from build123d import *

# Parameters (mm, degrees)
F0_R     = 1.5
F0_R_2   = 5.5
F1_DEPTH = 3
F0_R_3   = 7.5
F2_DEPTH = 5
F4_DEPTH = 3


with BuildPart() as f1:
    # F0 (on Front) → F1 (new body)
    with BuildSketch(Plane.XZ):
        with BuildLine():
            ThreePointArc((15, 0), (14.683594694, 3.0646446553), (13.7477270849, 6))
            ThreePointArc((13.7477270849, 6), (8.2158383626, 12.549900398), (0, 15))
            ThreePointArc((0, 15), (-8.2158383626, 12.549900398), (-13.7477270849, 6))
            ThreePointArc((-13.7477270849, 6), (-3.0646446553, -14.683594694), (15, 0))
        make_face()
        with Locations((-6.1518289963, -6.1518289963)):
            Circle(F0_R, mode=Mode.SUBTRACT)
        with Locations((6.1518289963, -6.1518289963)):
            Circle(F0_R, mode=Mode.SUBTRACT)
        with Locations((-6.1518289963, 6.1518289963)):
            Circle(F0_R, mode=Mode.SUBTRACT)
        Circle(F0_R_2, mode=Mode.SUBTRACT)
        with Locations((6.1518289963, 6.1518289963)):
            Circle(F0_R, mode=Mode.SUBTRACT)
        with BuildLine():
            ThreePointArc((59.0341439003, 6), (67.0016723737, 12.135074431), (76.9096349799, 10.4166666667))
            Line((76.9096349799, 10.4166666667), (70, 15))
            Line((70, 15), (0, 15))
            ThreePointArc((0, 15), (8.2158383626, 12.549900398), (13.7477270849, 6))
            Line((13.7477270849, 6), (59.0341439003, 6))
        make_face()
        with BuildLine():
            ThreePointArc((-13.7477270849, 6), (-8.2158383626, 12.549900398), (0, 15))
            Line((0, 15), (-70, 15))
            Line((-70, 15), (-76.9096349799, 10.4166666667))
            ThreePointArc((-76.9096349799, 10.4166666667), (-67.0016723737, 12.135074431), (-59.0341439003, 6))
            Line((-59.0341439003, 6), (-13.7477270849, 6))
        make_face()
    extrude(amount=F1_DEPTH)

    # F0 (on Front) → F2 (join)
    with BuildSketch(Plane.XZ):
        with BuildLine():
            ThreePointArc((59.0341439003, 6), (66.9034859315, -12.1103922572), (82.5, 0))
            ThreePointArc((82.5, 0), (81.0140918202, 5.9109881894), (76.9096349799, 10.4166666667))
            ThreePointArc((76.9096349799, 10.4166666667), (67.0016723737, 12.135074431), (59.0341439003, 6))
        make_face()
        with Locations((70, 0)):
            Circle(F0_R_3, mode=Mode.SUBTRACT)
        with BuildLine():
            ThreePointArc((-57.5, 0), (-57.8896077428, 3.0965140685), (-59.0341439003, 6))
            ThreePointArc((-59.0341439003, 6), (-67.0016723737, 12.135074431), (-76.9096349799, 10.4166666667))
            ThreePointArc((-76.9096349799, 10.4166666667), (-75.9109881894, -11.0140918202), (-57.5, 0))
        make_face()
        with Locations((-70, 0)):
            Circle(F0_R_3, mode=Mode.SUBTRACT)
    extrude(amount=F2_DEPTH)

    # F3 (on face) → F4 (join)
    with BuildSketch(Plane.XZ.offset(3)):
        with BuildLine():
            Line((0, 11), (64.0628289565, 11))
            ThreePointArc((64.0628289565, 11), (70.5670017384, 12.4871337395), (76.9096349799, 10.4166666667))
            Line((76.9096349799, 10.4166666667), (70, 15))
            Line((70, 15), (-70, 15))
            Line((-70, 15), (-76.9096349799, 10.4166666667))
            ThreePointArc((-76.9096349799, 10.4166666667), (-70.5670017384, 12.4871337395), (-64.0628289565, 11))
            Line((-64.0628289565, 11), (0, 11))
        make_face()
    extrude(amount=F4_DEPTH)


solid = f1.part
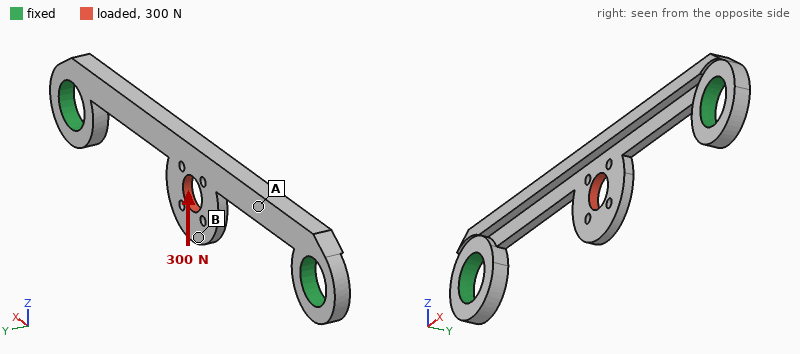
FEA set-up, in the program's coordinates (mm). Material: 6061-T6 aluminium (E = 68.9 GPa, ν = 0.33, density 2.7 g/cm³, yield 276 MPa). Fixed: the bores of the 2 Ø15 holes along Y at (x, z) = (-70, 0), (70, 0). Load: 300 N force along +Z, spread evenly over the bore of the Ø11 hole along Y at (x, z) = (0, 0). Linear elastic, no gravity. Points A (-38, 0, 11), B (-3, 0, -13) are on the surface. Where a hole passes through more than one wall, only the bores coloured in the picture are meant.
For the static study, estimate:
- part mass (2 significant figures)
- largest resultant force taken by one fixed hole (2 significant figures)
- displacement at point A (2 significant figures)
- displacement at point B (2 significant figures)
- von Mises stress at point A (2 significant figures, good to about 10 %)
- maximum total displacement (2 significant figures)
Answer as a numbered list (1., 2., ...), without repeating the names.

1. 26 g
2. 160 N
3. 0.078 mm
4. 0.19 mm
5. 16 MPa
6. 0.19 mm
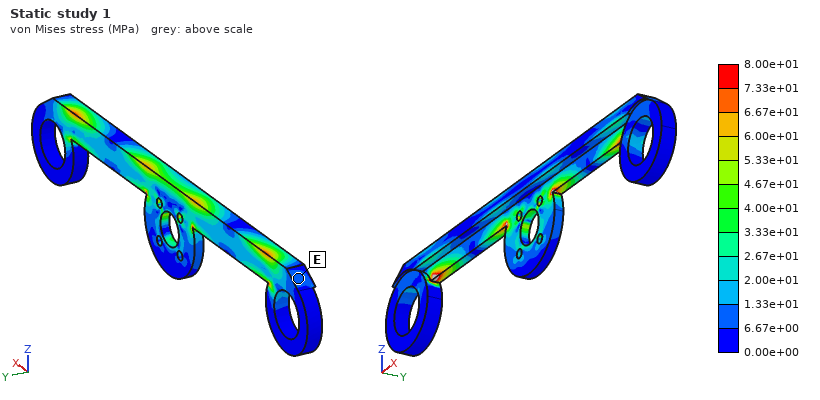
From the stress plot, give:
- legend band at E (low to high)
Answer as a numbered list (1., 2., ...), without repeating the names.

1. 6.67e+00 to 1.33e+01 MPa
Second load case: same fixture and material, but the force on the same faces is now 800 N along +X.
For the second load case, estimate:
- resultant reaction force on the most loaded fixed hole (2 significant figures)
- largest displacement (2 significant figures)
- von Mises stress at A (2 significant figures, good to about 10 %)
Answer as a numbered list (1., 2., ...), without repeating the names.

1. 410 N
2. 86 µm
3. 14 MPa
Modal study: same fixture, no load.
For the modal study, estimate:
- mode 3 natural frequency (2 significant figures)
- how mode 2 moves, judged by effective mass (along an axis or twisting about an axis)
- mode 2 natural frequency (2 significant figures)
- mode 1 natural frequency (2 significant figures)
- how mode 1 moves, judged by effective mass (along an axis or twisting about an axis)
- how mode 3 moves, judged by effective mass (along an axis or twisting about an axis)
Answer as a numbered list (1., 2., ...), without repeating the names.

1. 2600 Hz
2. along Z
3. 2100 Hz
4. 1100 Hz
5. along Y
6. along Z
